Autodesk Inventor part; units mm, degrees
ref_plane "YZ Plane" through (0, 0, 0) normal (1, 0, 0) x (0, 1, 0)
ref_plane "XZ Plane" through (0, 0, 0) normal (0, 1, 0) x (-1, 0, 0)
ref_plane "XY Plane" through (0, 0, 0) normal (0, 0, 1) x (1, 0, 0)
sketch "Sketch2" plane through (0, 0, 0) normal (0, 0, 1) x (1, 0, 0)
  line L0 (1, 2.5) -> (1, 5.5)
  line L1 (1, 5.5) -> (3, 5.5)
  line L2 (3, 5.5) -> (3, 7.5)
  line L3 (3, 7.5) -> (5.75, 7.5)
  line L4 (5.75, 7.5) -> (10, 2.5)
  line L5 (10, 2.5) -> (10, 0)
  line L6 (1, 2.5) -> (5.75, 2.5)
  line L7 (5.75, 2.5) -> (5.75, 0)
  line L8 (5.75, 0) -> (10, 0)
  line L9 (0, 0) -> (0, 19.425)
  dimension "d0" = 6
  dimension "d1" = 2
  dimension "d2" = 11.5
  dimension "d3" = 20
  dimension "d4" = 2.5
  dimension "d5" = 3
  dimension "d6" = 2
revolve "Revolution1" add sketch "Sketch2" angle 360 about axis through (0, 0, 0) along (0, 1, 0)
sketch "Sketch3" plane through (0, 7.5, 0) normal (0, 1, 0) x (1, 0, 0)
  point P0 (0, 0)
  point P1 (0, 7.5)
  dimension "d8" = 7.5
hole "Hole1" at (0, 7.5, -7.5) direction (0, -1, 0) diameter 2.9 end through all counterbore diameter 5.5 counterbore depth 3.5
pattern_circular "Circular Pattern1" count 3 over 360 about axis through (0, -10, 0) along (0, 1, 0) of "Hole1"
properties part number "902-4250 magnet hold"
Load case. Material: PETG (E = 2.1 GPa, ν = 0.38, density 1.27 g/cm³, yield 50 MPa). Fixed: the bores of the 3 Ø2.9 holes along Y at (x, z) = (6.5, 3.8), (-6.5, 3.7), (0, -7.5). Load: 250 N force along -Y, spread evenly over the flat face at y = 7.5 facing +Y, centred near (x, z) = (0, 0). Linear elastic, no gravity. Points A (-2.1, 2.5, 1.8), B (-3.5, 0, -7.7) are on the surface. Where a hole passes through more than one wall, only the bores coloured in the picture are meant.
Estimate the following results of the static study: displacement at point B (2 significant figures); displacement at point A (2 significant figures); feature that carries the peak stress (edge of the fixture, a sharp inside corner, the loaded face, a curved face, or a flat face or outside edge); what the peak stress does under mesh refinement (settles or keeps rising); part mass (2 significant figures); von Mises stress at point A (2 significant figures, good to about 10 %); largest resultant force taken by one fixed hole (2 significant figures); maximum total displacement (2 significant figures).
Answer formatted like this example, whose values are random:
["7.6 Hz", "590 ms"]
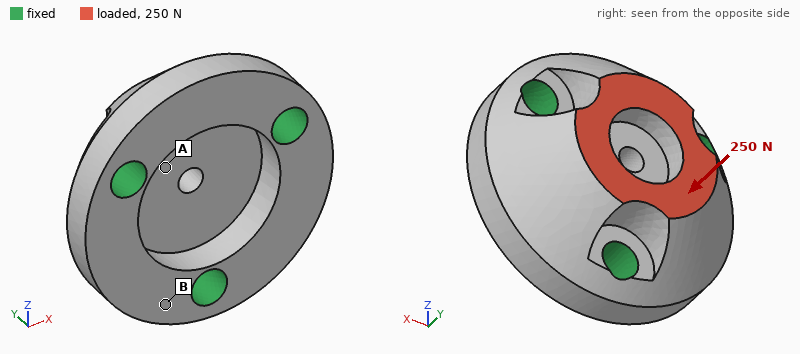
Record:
["7.0 µm", "21 µm", "edge of the fixture", "keeps rising", "1.6 g", "2.6 MPa", "89 N", "24 µm"]
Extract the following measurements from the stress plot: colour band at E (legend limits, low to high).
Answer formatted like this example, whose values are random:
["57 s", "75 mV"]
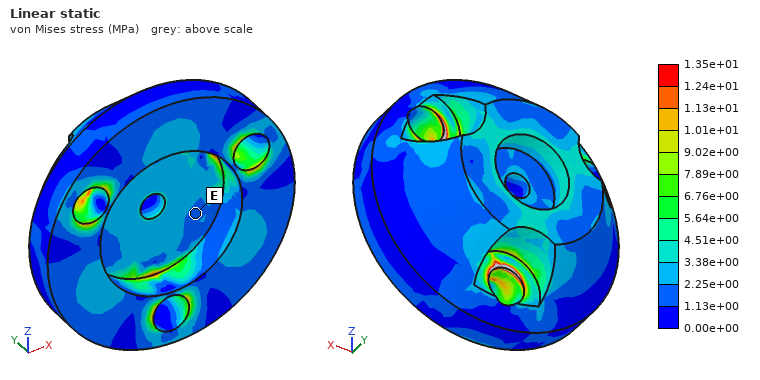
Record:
["1.13e+00 to 2.25e+00 MPa"]
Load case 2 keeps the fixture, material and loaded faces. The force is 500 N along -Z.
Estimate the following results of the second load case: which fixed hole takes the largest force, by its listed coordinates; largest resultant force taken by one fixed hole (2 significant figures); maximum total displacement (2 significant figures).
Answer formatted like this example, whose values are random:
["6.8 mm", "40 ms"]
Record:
["(0, -7.5)", "270 N", "95 µm"]
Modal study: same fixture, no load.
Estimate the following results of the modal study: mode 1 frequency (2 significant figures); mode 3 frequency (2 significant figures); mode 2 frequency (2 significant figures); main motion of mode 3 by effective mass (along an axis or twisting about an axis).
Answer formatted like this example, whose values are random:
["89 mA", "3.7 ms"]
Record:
["17 kHz", "18 kHz", "17 kHz", "along Y"]
